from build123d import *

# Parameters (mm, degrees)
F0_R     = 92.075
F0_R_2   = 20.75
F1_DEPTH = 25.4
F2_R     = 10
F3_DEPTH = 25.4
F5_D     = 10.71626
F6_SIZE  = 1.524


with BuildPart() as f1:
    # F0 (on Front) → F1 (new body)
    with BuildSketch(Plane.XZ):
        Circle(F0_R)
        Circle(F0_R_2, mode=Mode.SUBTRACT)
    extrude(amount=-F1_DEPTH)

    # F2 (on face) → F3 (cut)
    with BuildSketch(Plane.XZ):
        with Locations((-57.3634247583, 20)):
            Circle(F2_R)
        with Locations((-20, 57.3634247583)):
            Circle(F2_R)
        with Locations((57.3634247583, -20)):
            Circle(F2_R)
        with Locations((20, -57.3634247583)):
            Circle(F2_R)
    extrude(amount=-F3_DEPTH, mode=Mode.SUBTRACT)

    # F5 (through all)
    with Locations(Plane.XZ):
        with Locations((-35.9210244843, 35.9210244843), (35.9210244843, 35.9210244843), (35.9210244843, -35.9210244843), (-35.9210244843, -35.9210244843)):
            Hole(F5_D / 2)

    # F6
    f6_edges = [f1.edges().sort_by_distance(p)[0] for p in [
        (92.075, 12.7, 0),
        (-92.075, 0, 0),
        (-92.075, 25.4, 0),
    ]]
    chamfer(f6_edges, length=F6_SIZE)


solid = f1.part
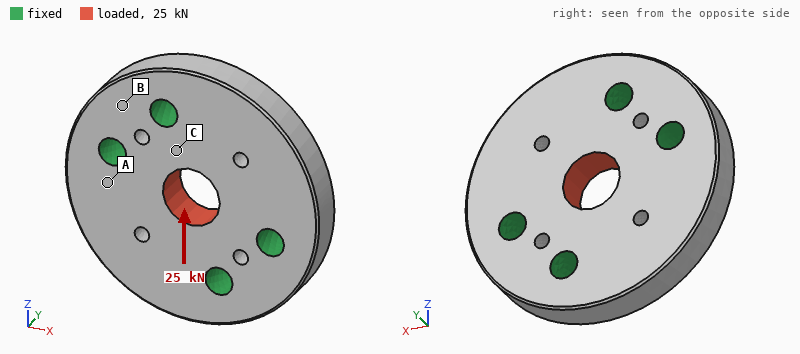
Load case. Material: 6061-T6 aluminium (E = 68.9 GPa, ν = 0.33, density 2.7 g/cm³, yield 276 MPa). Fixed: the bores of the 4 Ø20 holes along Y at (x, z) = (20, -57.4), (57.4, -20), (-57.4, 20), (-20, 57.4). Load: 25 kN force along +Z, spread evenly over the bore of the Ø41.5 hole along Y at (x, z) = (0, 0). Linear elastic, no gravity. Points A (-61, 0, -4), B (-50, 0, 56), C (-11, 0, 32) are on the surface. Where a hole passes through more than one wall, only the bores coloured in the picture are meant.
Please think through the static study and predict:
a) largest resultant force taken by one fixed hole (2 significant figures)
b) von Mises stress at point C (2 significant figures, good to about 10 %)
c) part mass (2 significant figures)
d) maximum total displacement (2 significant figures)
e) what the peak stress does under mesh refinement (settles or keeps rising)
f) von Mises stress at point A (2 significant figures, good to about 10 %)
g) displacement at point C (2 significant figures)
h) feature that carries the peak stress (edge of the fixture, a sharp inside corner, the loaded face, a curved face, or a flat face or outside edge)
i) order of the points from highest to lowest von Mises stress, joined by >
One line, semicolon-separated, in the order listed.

8.0 kN; 9.0 MPa; 1.6 kg; 6.1 µm; keeps rising; 3.0 MPa; 2.9 µm; edge of the fixture; C > A > B
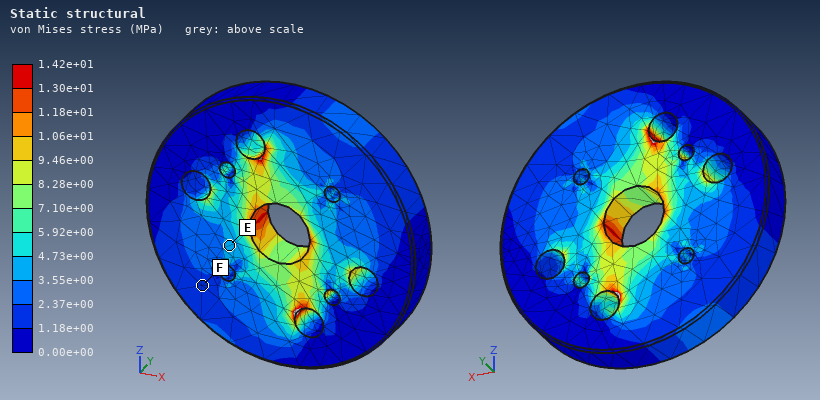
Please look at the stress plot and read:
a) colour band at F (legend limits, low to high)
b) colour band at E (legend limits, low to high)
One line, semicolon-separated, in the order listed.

1.18e+00 to 2.37e+00 MPa; 3.55e+00 to 4.73e+00 MPa
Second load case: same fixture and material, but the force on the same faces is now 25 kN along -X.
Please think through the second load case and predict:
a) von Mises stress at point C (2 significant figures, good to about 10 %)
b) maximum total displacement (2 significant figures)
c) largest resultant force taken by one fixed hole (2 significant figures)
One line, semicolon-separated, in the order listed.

5.3 MPa; 6.1 µm; 8.0 kN
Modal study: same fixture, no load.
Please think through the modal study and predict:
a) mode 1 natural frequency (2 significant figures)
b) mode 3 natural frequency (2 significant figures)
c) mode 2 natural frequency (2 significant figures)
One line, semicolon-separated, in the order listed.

4800 Hz; 10 kHz; 4900 Hz
